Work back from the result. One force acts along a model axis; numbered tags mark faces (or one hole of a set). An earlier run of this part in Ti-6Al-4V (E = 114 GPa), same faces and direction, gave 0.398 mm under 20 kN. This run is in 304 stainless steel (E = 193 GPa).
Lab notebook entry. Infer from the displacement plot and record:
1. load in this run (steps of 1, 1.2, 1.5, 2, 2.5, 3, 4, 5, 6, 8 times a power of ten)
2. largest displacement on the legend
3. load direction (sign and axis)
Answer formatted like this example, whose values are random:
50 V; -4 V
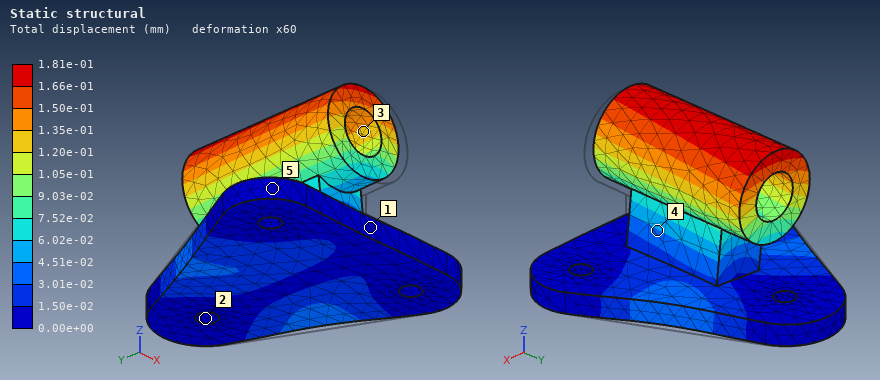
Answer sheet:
15 kN; 1.81e-01 mm; -X
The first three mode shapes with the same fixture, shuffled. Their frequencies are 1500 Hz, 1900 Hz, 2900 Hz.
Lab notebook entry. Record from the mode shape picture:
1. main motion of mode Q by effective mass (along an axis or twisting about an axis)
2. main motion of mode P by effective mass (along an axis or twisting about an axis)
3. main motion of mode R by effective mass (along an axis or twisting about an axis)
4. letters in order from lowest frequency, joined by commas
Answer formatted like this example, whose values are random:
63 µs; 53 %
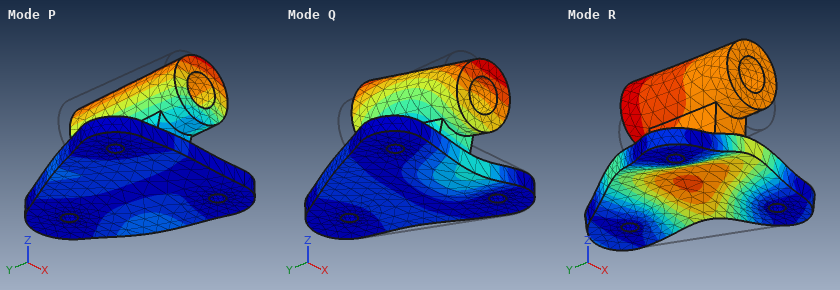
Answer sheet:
along Y; along X; along Z; P, Q, R
